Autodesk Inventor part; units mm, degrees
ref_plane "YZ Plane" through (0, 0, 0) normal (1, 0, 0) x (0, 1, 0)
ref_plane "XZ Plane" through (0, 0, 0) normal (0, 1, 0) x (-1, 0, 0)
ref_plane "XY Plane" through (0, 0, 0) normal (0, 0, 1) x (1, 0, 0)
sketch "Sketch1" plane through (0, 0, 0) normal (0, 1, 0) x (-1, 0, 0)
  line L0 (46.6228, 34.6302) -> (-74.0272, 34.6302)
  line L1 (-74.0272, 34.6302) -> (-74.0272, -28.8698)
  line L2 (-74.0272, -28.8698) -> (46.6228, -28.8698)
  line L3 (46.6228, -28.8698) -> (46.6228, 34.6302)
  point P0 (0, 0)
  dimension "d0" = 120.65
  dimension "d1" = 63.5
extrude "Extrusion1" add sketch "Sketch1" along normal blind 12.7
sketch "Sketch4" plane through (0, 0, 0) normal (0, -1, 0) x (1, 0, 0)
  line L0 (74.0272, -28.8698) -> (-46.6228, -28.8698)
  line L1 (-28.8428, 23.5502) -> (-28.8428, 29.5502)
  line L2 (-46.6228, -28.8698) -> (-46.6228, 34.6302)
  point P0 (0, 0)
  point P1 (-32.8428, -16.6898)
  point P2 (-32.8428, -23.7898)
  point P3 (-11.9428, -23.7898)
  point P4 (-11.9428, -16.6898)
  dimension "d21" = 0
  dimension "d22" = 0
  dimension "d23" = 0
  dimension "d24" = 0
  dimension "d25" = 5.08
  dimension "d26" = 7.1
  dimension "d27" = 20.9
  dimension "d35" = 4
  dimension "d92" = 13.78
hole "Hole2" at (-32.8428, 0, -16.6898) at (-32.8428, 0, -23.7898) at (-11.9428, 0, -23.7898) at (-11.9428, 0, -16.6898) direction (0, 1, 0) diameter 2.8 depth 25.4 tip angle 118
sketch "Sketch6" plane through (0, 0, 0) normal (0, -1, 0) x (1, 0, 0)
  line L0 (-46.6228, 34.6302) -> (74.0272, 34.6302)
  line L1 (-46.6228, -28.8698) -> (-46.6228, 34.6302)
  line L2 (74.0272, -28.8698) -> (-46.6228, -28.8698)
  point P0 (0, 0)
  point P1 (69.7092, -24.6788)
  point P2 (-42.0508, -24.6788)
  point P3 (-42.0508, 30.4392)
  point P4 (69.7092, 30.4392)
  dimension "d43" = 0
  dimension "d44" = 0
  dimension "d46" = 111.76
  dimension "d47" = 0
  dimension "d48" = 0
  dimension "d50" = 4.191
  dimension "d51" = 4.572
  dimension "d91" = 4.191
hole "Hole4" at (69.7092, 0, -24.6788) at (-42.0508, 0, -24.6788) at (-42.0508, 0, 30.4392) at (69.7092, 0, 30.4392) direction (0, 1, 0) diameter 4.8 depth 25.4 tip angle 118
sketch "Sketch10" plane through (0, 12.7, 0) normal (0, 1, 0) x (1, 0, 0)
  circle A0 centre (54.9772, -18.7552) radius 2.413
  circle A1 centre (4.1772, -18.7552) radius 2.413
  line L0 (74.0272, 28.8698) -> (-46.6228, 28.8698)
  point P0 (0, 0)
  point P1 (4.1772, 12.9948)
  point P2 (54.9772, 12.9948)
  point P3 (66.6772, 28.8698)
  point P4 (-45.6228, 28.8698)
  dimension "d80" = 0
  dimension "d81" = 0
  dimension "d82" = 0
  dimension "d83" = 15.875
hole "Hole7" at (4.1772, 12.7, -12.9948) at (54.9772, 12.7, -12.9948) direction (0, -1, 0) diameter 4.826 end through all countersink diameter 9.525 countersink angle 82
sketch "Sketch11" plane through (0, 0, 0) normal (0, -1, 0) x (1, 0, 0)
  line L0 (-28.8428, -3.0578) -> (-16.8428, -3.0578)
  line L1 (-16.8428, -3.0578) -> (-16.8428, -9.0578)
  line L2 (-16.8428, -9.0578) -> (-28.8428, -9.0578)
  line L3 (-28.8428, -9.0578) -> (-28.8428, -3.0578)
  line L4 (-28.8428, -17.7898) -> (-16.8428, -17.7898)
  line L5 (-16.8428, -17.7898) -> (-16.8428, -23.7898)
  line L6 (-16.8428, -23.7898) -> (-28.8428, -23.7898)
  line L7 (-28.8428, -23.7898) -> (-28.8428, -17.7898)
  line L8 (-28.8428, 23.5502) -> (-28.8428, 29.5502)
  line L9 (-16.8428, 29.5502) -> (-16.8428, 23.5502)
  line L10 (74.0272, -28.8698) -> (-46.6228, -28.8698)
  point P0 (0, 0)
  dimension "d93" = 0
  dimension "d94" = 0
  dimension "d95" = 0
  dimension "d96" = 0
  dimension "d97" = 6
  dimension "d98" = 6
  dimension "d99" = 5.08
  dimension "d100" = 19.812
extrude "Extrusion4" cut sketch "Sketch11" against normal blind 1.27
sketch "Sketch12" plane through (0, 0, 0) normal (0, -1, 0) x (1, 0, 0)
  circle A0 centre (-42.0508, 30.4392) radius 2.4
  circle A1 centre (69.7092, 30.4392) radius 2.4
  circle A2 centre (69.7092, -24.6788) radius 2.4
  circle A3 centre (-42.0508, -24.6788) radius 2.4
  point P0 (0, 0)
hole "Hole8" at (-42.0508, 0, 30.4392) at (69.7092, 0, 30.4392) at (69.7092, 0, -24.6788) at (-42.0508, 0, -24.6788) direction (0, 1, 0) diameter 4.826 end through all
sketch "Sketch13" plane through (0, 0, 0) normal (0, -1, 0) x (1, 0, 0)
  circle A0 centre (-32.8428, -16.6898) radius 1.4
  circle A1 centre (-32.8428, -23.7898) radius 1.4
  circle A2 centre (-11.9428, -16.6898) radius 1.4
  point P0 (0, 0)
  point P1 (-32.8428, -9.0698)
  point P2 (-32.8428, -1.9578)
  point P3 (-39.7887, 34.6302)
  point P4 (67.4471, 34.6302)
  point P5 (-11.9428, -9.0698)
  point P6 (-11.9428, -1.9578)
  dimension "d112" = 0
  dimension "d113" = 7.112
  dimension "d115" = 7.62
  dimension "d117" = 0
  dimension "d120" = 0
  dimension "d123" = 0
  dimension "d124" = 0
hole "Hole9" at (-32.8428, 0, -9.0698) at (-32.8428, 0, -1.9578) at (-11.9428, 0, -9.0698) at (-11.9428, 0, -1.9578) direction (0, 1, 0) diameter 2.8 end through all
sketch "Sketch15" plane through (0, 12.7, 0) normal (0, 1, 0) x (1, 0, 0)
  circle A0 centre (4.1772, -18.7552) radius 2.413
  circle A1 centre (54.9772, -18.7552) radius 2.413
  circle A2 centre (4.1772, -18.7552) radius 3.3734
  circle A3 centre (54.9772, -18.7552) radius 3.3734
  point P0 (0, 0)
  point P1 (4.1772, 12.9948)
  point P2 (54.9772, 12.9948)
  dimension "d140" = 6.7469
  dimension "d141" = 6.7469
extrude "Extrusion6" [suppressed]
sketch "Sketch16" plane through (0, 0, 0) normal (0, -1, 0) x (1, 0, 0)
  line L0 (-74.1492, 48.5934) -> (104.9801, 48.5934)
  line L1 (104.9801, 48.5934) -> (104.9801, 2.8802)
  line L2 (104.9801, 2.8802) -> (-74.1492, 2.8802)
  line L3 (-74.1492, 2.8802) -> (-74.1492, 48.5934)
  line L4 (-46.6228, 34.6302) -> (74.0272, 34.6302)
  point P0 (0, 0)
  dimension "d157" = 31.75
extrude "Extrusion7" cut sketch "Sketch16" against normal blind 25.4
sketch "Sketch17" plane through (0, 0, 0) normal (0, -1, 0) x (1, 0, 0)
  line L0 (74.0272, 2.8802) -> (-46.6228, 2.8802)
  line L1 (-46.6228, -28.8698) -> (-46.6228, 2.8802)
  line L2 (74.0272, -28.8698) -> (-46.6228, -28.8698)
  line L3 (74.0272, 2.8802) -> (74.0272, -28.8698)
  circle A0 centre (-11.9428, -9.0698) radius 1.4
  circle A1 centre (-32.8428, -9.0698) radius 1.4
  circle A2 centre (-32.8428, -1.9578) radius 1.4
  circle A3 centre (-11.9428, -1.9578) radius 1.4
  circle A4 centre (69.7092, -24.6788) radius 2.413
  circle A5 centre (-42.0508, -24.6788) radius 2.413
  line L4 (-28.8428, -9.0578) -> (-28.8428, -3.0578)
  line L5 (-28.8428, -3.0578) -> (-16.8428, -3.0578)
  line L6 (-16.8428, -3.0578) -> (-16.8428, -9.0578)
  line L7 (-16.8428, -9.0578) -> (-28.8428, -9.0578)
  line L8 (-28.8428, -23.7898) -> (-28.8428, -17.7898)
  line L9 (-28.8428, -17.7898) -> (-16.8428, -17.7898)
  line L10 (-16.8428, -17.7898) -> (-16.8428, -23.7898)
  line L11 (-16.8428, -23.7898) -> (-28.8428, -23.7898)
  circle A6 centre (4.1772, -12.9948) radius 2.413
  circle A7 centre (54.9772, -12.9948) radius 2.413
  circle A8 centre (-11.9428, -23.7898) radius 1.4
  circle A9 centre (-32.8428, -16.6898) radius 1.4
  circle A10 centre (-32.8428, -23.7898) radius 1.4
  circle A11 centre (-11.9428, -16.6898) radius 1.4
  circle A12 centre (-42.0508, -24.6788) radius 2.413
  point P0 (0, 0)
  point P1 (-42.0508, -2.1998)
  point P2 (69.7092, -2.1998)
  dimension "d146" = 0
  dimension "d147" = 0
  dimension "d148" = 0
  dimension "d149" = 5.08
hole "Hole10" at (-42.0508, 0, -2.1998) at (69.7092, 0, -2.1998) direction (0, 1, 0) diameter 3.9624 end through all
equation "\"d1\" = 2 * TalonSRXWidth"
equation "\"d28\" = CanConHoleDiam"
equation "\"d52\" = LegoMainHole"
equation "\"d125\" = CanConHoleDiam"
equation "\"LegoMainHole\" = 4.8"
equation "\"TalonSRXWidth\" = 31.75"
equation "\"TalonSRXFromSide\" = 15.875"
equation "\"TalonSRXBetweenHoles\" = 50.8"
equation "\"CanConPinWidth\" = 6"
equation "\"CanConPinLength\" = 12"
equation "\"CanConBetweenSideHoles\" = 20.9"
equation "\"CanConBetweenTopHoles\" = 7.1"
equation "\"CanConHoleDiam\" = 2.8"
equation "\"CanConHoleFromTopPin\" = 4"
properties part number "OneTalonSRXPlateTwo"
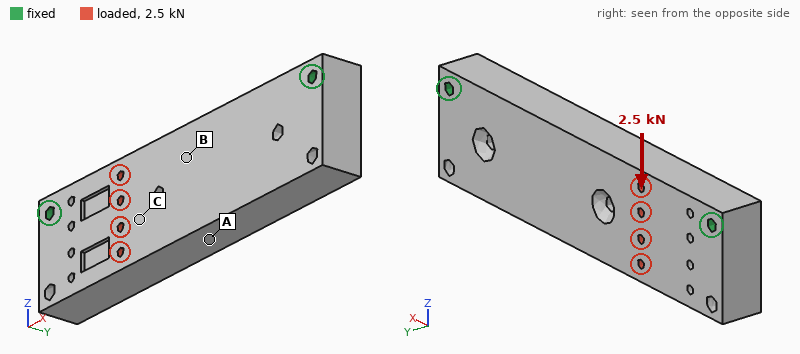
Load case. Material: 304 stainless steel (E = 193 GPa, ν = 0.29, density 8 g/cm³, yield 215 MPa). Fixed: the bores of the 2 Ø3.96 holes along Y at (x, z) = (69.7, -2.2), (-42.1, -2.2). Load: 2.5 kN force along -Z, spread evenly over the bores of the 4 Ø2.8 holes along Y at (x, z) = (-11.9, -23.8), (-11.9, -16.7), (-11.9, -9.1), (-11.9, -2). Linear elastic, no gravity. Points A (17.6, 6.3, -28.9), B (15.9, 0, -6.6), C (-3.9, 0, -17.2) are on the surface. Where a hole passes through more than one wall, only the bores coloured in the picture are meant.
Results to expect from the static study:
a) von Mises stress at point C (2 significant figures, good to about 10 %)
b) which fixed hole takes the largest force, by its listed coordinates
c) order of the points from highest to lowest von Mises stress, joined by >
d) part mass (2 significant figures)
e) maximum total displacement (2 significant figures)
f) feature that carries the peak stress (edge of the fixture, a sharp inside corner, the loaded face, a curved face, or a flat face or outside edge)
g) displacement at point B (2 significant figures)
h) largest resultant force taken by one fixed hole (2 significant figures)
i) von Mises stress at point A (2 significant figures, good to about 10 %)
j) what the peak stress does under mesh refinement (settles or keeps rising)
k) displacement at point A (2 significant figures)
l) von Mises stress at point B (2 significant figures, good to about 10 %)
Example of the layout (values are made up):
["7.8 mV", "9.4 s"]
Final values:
["6.2 MPa", "(-42.1, -2.2)", "A > C > B", "370 g", "6.7 µm", "edge of the fixture", "5.8 µm", "2.2 kN", "11 MPa", "keeps rising", "5.5 µm", "3.6 MPa"]
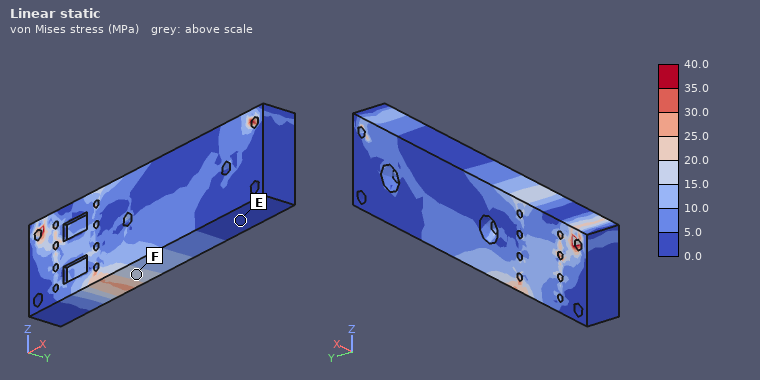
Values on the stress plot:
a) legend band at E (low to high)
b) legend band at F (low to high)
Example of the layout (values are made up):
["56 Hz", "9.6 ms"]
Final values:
["0.0 to 5.0 MPa", "15.0 to 20.0 MPa"]
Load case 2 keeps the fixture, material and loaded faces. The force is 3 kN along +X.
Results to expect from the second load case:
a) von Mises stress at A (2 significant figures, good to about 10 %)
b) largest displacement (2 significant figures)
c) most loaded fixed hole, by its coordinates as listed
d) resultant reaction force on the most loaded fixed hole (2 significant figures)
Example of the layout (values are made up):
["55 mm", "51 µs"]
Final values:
["3.6 MPa", "2.2 µm", "(-42.1, -2.2)", "1.8 kN"]
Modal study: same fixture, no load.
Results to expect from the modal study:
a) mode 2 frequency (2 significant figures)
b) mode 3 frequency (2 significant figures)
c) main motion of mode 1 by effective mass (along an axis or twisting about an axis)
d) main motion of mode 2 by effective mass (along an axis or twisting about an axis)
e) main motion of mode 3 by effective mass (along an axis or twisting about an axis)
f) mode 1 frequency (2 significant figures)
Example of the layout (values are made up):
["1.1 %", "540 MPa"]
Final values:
["6500 Hz", "6800 Hz", "along Y", "along Z", "twisting about X", "3400 Hz"]
